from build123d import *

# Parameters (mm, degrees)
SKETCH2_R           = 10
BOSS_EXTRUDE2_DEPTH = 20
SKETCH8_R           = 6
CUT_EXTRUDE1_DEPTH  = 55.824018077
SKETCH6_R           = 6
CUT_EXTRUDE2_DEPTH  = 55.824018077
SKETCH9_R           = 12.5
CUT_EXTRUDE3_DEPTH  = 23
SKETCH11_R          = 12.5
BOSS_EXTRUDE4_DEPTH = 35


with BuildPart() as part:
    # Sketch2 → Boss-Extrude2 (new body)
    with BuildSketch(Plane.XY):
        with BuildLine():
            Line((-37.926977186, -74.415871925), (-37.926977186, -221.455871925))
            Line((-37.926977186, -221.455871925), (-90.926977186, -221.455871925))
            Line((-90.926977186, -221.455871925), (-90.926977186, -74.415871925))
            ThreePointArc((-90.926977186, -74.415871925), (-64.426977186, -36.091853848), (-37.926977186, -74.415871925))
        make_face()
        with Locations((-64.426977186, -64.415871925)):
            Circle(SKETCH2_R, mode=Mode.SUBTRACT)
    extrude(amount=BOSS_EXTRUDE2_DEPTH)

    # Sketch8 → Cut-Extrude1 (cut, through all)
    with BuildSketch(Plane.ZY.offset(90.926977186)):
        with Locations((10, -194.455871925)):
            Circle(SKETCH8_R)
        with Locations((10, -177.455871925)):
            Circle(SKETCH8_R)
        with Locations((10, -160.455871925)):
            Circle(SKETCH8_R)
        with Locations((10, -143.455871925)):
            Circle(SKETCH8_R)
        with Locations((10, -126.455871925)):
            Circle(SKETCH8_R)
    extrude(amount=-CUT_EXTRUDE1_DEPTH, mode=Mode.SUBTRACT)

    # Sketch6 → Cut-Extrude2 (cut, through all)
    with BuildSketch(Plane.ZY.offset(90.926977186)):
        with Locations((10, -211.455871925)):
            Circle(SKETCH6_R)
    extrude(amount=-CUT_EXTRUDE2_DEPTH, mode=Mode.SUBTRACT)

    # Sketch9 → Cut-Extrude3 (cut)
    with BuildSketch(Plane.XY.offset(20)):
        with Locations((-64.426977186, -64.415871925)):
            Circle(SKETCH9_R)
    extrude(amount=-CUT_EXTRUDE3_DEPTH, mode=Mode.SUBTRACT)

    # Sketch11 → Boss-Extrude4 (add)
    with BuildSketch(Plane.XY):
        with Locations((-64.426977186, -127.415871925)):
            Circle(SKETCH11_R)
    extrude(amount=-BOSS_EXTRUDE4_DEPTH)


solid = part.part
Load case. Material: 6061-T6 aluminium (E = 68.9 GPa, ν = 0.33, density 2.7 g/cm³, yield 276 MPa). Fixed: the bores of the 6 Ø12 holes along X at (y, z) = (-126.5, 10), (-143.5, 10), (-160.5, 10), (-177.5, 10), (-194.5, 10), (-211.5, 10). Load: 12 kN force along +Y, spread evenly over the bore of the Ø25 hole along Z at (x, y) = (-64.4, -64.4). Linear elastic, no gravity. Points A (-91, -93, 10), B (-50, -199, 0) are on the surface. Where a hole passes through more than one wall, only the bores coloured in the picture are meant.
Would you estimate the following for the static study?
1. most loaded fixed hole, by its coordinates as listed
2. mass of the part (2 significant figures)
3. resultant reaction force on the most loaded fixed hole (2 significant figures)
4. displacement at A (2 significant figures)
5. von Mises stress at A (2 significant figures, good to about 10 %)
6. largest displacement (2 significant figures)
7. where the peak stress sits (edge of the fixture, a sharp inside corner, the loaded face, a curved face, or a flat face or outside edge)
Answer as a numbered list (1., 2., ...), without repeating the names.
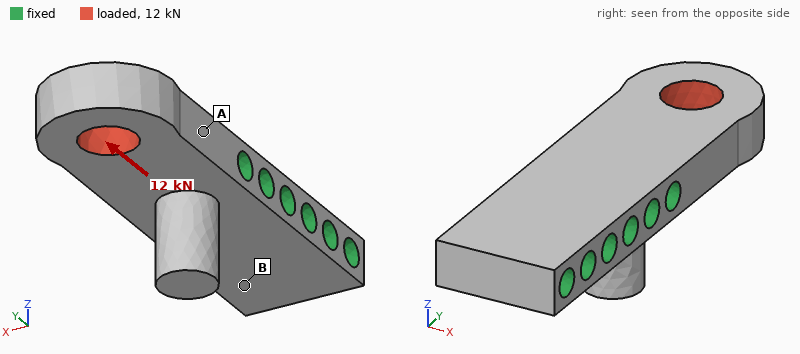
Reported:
1. (-126.5, 10)
2. 440 g
3. 11 kN
4. 5.7 µm
5. 14 MPa
6. 18 µm
7. the loaded face
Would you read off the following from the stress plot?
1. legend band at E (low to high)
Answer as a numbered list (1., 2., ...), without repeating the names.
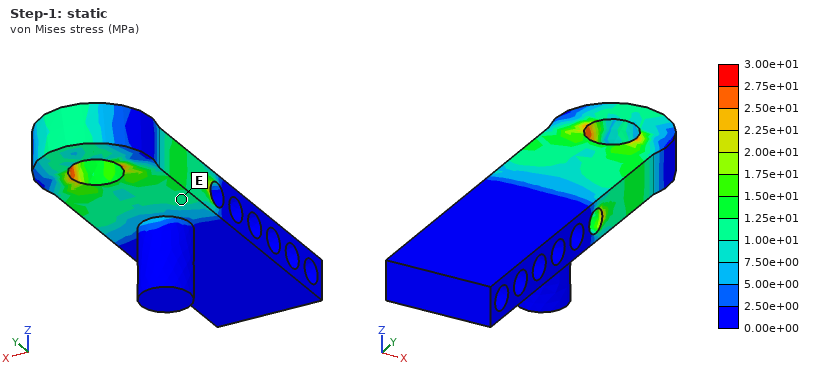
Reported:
1. 1.00e+01 to 1.25e+01 MPa
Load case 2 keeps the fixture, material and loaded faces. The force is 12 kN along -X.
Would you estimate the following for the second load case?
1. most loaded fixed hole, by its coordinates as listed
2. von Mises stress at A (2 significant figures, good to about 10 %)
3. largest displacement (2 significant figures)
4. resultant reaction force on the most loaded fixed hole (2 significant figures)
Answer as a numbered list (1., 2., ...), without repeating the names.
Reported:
1. (-126.5, 10)
2. 42 MPa
3. 0.13 mm
4. 12 kN
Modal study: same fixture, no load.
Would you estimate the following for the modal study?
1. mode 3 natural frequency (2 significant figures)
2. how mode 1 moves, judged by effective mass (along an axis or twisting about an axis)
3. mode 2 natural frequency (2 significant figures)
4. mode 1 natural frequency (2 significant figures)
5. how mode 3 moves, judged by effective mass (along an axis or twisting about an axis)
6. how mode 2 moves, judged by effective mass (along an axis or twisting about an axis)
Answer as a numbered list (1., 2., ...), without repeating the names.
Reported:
1. 6300 Hz
2. along Z
3. 5100 Hz
4. 2400 Hz
5. twisting about Y
6. along X
